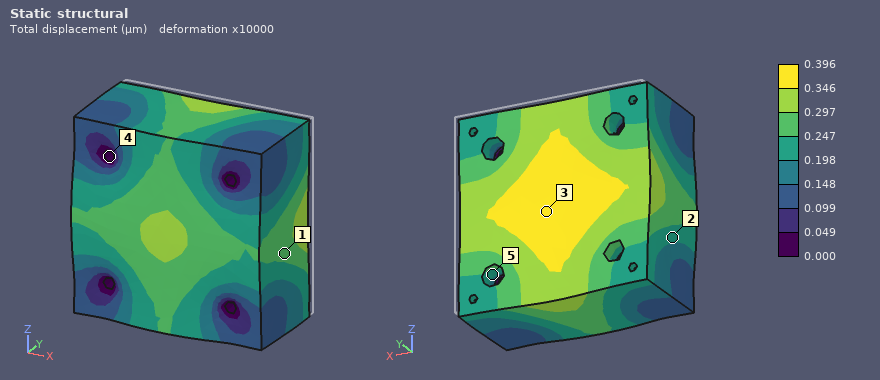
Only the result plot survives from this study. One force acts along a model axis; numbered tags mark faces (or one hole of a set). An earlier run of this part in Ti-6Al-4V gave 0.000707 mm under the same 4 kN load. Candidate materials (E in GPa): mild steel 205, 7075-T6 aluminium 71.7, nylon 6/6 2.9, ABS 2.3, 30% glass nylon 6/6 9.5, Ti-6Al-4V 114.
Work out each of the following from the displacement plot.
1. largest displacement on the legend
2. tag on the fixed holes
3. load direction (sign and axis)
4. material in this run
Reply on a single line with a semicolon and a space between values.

0.396 µm; 4; -Y; mild steel
